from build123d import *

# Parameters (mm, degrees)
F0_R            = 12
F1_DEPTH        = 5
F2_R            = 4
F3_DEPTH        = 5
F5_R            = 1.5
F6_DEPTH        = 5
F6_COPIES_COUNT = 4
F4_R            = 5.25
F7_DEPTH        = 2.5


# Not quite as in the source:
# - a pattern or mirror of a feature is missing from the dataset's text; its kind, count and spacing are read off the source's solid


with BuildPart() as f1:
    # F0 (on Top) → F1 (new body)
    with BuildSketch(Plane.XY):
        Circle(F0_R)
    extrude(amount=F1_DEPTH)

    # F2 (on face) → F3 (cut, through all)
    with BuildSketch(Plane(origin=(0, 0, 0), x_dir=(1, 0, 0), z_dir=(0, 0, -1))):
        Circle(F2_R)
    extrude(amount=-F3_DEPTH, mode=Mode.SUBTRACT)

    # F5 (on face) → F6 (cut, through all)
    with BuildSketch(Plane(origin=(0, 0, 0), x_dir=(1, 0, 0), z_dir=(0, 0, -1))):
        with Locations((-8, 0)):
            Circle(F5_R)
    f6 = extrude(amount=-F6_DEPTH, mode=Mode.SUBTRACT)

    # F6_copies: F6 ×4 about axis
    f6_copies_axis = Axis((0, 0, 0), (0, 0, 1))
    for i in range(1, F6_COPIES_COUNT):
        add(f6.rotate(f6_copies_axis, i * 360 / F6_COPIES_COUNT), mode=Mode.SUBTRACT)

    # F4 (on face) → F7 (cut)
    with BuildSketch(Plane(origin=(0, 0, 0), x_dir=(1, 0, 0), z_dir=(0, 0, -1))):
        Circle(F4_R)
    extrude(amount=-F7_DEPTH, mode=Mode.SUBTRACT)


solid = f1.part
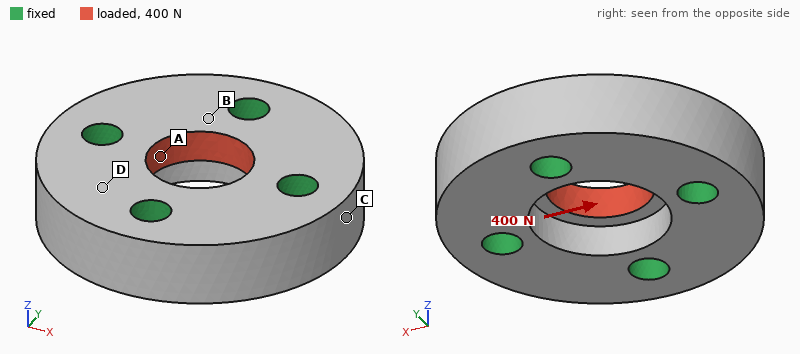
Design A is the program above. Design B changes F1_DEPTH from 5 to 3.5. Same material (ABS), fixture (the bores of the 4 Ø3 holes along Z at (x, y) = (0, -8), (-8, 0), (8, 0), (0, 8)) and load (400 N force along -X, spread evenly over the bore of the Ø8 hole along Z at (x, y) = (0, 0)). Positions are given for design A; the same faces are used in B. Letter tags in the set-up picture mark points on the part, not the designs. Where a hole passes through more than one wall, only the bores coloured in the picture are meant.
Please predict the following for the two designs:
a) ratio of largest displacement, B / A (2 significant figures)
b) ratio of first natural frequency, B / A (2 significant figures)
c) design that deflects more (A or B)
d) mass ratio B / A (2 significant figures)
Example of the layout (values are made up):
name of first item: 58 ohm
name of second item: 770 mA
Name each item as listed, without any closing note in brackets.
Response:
ratio of largest displacement, B / A: 2.1
ratio of first natural frequency, B / A: 0.84
design that deflects more: B
mass ratio B / A: 0.68
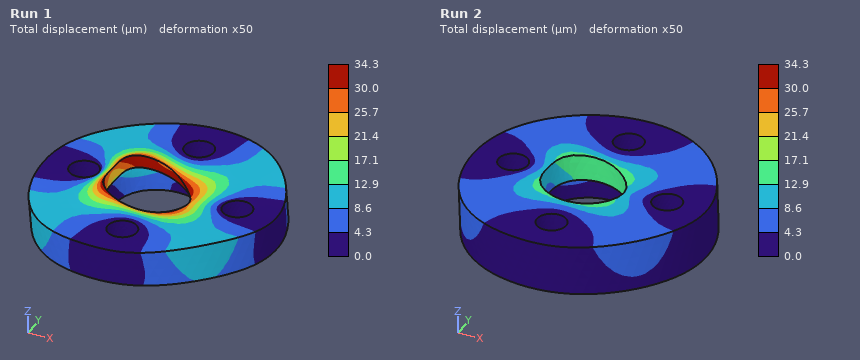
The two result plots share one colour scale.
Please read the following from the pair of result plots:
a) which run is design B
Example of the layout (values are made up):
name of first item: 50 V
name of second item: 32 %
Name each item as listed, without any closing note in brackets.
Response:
which run is design B: Run 1
